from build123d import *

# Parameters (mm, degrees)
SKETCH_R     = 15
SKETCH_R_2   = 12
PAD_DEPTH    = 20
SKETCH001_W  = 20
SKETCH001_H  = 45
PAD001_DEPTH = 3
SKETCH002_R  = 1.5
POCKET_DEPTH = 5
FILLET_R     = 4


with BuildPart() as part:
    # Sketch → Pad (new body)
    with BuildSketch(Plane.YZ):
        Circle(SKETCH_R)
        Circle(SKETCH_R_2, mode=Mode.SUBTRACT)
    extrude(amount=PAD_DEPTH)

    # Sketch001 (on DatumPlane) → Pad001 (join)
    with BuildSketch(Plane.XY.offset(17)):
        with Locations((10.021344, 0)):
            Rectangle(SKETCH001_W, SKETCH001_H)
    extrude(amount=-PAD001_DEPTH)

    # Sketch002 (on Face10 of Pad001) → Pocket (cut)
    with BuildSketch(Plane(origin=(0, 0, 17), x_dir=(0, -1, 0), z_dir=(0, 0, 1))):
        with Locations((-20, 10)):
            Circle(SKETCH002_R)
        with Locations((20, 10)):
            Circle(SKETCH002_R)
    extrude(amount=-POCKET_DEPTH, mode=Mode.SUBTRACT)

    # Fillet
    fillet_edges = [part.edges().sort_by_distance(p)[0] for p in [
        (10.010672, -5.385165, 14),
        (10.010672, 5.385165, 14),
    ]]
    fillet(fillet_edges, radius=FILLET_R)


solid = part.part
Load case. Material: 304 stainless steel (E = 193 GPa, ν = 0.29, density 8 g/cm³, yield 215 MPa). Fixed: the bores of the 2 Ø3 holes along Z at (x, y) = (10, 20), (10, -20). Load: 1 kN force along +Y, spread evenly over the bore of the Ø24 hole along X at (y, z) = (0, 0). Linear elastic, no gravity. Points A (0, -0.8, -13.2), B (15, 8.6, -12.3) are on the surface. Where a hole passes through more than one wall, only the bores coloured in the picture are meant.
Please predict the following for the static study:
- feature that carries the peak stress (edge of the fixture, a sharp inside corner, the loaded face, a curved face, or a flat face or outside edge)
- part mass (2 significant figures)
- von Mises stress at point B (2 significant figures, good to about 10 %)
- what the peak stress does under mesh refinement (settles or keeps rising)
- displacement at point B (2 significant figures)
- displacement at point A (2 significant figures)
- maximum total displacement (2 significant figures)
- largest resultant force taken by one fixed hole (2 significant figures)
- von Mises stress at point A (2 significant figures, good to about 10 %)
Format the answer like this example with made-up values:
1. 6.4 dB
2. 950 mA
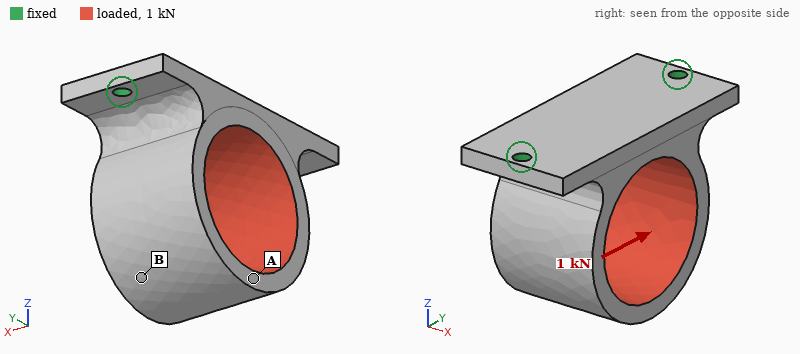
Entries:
1. edge of the fixture
2. 66 g
3. 30 MPa
4. keeps rising
5. 33 µm
6. 33 µm
7. 33 µm
8. 670 N
9. 13 MPa
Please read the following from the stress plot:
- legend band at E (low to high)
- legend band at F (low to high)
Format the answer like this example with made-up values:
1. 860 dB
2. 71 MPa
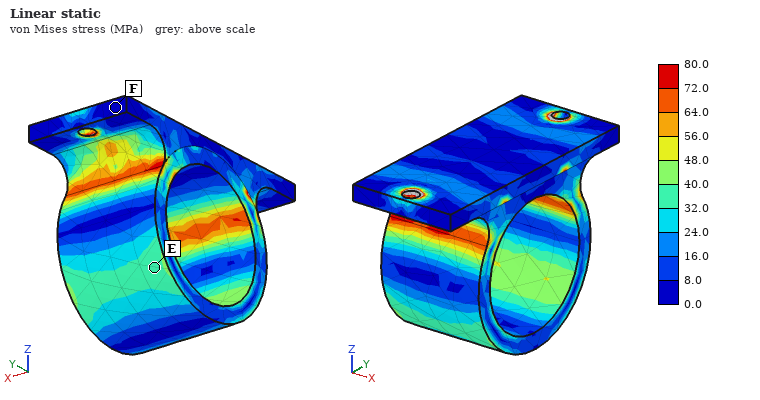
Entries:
1. 32.0 to 40.0 MPa
2. 0.0 to 8.0 MPa
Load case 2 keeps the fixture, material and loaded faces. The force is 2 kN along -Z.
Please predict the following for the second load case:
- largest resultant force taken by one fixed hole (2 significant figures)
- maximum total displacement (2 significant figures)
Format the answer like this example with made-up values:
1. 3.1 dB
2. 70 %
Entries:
1. 1.2 kN
2. 16 µm
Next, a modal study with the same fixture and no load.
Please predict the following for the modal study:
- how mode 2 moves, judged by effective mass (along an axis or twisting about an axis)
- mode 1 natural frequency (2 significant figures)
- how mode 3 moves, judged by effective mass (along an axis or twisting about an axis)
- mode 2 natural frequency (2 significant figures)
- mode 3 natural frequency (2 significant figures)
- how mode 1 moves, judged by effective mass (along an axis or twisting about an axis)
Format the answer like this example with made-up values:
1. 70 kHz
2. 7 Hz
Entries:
1. along Y
2. 2300 Hz
3. along Z
4. 4700 Hz
5. 8000 Hz
6. along X
